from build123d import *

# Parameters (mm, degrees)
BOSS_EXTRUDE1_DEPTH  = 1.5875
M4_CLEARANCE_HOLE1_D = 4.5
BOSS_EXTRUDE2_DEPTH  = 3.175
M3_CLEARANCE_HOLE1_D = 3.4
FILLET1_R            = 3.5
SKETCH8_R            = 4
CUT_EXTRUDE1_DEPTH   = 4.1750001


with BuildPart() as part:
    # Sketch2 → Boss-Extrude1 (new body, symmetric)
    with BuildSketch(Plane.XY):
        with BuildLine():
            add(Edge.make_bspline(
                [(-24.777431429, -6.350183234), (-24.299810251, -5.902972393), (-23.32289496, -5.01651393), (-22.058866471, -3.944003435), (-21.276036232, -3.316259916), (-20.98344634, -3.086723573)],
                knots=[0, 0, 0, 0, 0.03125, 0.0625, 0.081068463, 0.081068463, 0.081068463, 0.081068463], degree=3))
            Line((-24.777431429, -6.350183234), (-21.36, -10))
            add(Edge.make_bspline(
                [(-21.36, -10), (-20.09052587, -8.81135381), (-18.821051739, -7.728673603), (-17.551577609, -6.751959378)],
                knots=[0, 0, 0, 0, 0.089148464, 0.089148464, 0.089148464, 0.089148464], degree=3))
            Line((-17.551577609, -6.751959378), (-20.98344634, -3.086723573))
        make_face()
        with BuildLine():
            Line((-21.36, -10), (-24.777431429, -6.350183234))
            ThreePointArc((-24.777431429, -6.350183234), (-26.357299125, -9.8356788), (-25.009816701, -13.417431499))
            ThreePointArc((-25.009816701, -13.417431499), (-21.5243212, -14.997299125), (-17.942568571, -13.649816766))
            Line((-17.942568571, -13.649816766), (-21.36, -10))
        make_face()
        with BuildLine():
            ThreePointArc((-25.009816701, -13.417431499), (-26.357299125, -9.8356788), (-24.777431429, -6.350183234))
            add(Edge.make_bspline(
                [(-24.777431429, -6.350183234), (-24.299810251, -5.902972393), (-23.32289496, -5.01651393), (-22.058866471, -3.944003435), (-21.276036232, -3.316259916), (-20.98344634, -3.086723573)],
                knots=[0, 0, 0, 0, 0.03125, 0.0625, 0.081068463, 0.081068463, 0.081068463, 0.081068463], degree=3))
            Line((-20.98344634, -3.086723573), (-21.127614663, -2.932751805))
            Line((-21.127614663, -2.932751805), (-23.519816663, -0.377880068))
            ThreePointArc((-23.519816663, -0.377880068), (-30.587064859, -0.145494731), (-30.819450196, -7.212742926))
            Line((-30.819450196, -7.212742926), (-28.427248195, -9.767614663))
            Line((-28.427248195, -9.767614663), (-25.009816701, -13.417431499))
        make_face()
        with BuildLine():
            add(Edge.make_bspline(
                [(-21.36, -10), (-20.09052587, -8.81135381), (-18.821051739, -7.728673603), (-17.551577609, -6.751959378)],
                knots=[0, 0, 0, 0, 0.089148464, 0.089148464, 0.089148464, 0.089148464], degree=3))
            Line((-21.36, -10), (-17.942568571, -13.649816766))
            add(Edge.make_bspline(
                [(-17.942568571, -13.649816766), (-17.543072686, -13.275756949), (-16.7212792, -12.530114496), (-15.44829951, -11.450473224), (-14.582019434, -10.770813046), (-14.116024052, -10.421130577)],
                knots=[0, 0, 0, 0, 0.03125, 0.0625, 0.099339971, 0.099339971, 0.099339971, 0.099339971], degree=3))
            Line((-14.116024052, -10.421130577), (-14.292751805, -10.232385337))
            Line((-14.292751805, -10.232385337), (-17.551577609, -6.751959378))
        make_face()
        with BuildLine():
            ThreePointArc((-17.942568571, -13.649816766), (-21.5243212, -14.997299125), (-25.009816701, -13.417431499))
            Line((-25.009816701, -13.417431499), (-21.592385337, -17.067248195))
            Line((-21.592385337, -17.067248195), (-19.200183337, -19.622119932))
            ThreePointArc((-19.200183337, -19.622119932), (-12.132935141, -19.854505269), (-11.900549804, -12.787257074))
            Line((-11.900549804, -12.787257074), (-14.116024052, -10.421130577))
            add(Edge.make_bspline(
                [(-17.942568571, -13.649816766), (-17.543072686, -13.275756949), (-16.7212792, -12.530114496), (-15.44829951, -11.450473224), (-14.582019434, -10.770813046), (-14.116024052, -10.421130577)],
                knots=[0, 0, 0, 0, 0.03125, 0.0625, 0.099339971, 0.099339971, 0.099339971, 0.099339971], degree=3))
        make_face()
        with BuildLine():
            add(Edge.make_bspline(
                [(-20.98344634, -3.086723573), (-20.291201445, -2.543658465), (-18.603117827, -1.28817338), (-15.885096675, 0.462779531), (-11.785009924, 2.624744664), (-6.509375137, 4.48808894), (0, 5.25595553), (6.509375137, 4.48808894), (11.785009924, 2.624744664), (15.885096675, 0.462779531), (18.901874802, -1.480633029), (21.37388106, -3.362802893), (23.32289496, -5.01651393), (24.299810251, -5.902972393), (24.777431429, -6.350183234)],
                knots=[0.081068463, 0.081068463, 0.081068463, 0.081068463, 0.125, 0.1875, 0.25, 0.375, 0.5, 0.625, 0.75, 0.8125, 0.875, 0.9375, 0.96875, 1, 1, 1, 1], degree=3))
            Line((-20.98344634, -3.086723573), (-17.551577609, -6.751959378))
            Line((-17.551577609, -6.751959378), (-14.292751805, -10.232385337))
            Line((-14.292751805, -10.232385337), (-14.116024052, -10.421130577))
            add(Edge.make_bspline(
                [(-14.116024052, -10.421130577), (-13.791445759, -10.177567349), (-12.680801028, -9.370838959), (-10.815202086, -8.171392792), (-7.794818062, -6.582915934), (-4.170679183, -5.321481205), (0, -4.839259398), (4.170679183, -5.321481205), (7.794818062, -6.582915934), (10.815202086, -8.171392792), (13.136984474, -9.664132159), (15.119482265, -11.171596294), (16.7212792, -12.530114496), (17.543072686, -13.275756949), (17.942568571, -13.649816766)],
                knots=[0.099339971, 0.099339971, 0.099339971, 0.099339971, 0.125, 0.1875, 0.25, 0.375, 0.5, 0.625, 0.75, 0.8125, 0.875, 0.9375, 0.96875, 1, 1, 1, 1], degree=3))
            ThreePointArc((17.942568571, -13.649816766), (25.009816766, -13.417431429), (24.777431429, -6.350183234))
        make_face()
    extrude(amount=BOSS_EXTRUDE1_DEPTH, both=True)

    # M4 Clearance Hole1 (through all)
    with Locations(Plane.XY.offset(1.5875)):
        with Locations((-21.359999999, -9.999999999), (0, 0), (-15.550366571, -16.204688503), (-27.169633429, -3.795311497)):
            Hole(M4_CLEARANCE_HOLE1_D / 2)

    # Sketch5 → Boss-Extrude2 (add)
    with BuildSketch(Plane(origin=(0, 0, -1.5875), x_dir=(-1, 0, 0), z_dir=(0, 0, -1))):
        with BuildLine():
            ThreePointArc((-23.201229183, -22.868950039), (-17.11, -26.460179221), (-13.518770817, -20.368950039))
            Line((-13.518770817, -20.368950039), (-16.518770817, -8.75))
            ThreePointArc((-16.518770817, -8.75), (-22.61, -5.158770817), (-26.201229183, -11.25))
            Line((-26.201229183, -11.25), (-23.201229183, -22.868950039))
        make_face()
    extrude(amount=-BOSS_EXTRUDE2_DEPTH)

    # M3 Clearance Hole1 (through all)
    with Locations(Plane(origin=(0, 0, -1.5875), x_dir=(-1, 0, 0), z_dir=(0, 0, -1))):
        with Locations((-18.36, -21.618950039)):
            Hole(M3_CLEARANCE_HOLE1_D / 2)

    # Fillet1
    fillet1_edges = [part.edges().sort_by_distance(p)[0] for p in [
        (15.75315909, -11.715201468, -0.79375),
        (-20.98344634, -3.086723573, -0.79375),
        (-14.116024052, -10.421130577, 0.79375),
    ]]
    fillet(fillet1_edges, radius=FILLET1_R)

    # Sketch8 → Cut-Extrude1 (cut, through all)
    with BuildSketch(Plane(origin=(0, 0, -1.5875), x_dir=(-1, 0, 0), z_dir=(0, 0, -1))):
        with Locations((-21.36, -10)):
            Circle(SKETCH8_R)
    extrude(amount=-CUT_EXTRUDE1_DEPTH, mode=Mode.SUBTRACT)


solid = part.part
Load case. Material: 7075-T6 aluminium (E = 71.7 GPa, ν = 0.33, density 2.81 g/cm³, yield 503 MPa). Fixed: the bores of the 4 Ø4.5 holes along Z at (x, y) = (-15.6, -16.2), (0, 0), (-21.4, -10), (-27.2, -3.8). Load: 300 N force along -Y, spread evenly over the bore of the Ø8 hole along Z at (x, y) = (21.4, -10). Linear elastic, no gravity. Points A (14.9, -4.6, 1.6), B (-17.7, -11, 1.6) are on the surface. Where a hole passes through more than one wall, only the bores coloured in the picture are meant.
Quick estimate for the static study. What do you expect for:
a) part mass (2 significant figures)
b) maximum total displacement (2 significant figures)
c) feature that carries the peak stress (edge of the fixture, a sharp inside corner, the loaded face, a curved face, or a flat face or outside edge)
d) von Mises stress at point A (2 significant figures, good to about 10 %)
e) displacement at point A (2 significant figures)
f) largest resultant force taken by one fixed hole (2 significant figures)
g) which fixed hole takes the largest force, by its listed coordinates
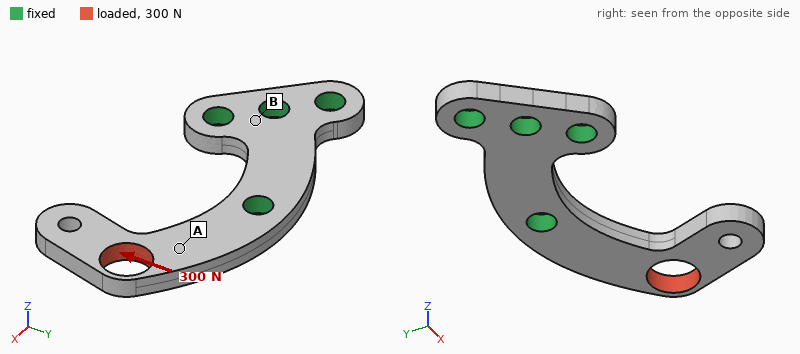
6.5 g
0.17 mm
edge of the fixture
26 MPa
0.043 mm
390 N
(0, 0)
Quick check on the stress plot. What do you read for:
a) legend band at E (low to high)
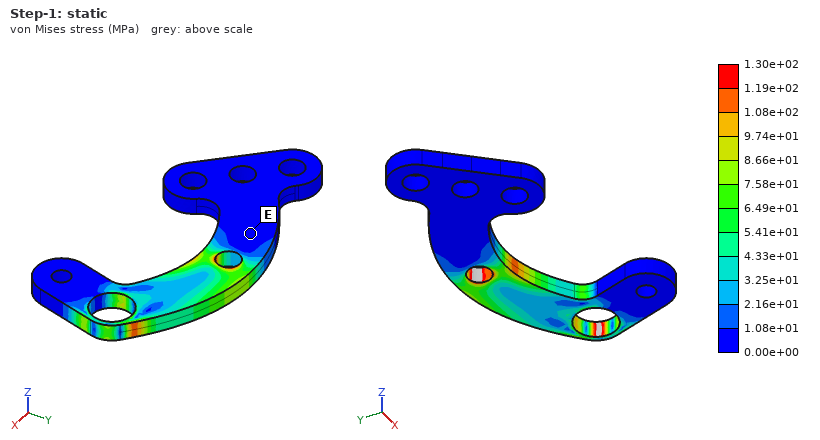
0.00e+00 to 1.08e+01 MPa
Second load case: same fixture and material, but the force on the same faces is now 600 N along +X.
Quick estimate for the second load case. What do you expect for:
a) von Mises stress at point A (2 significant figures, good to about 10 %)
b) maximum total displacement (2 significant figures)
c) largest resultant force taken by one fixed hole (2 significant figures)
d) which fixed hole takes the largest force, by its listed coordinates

37 MPa
0.20 mm
580 N
(0, 0)
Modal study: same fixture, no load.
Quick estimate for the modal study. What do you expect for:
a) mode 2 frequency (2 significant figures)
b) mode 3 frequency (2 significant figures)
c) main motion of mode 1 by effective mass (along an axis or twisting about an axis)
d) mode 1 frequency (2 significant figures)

5300 Hz
6700 Hz
along Z
2300 Hz
